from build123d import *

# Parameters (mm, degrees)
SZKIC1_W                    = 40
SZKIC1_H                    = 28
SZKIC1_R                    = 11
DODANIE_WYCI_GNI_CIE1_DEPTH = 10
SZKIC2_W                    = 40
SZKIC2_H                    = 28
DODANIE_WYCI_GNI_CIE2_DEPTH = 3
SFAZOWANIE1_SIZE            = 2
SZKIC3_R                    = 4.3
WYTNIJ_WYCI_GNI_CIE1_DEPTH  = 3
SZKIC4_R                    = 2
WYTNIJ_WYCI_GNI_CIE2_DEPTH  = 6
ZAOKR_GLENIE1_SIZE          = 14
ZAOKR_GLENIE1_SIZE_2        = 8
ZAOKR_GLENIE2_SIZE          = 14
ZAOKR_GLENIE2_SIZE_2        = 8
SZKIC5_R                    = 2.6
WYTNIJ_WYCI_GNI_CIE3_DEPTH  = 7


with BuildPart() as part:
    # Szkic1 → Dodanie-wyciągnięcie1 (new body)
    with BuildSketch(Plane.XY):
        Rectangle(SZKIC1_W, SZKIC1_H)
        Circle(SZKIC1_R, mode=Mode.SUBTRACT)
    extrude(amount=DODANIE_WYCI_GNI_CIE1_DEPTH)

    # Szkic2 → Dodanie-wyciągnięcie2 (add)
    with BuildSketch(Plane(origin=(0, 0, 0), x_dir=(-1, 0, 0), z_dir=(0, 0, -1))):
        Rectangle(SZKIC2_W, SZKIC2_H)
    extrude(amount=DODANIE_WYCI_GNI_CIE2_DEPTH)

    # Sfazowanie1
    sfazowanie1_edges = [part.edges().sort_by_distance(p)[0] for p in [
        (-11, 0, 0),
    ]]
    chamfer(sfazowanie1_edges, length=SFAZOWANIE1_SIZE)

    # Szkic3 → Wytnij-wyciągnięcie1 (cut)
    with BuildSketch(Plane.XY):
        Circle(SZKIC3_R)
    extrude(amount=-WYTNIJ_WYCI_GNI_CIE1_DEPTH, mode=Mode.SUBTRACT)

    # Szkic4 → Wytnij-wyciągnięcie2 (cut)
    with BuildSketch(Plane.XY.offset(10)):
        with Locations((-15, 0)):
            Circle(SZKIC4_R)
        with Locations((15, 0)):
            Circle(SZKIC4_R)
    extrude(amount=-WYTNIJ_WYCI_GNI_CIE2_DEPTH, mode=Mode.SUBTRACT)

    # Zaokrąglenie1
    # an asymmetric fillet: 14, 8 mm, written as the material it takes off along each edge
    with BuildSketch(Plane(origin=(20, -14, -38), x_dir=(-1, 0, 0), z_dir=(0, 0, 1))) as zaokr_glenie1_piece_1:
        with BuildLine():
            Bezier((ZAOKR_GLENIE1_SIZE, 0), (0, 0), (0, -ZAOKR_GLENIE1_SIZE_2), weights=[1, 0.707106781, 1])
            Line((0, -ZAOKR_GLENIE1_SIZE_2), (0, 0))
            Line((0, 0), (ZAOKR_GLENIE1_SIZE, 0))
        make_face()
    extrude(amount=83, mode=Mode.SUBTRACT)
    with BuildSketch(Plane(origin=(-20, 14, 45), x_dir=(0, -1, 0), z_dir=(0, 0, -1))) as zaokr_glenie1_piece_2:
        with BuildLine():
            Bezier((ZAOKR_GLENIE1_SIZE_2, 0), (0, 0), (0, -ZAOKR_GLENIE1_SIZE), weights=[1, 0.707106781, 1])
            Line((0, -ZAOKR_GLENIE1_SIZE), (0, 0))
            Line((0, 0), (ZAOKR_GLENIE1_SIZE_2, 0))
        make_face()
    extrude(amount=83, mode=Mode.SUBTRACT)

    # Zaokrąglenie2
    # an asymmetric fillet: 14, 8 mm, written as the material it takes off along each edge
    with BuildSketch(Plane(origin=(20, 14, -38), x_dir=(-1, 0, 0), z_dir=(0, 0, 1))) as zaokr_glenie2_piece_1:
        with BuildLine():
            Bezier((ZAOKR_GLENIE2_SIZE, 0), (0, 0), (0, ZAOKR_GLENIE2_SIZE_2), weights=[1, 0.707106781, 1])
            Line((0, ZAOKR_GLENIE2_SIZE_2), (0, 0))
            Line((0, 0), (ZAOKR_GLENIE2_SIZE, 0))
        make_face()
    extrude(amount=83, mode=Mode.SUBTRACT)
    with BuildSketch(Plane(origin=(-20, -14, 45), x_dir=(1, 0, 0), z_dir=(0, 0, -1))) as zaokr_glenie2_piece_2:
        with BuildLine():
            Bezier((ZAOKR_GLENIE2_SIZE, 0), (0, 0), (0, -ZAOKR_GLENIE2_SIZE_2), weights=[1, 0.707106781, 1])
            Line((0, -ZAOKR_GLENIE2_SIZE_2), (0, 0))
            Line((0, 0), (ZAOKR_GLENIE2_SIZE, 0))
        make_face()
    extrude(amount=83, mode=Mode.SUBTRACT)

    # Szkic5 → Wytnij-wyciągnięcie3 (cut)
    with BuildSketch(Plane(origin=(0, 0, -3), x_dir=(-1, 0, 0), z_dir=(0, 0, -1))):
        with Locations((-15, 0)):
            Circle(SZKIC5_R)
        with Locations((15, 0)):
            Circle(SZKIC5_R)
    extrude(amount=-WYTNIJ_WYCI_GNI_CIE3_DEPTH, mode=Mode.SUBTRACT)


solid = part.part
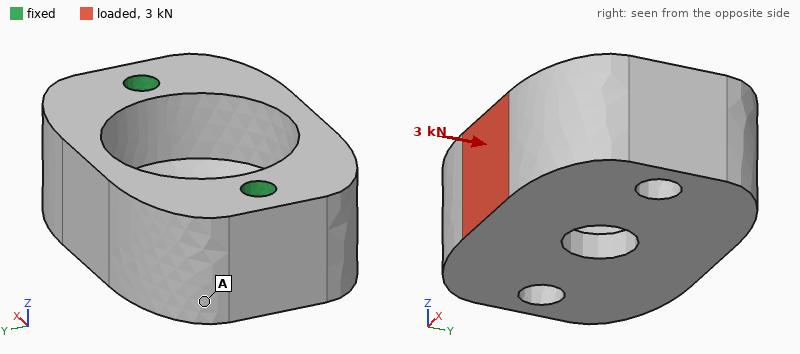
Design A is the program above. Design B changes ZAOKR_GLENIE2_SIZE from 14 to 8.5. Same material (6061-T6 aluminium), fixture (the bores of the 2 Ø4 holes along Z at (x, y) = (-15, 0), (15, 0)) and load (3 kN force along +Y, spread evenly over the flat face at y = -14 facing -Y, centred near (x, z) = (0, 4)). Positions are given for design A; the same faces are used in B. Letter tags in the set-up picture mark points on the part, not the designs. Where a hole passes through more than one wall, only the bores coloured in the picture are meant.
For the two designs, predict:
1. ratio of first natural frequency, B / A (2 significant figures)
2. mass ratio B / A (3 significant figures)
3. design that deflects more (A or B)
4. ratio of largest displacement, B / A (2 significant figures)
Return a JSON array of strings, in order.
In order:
["0.98", "1.03", "A", "0.77"]
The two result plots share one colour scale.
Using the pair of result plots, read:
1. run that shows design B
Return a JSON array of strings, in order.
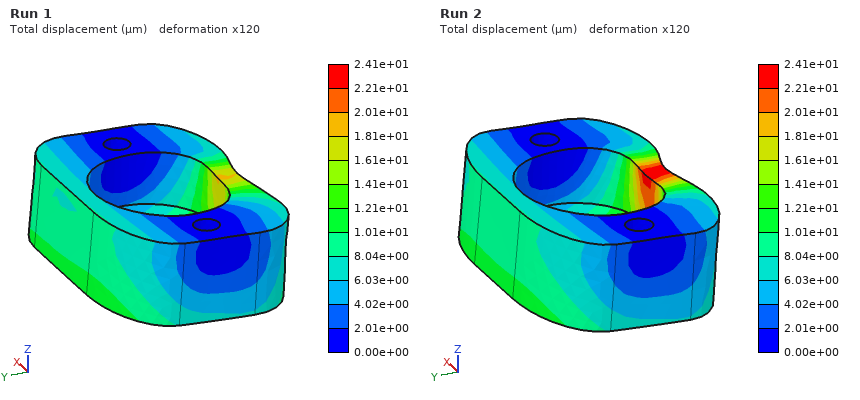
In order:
["Run 1"]
